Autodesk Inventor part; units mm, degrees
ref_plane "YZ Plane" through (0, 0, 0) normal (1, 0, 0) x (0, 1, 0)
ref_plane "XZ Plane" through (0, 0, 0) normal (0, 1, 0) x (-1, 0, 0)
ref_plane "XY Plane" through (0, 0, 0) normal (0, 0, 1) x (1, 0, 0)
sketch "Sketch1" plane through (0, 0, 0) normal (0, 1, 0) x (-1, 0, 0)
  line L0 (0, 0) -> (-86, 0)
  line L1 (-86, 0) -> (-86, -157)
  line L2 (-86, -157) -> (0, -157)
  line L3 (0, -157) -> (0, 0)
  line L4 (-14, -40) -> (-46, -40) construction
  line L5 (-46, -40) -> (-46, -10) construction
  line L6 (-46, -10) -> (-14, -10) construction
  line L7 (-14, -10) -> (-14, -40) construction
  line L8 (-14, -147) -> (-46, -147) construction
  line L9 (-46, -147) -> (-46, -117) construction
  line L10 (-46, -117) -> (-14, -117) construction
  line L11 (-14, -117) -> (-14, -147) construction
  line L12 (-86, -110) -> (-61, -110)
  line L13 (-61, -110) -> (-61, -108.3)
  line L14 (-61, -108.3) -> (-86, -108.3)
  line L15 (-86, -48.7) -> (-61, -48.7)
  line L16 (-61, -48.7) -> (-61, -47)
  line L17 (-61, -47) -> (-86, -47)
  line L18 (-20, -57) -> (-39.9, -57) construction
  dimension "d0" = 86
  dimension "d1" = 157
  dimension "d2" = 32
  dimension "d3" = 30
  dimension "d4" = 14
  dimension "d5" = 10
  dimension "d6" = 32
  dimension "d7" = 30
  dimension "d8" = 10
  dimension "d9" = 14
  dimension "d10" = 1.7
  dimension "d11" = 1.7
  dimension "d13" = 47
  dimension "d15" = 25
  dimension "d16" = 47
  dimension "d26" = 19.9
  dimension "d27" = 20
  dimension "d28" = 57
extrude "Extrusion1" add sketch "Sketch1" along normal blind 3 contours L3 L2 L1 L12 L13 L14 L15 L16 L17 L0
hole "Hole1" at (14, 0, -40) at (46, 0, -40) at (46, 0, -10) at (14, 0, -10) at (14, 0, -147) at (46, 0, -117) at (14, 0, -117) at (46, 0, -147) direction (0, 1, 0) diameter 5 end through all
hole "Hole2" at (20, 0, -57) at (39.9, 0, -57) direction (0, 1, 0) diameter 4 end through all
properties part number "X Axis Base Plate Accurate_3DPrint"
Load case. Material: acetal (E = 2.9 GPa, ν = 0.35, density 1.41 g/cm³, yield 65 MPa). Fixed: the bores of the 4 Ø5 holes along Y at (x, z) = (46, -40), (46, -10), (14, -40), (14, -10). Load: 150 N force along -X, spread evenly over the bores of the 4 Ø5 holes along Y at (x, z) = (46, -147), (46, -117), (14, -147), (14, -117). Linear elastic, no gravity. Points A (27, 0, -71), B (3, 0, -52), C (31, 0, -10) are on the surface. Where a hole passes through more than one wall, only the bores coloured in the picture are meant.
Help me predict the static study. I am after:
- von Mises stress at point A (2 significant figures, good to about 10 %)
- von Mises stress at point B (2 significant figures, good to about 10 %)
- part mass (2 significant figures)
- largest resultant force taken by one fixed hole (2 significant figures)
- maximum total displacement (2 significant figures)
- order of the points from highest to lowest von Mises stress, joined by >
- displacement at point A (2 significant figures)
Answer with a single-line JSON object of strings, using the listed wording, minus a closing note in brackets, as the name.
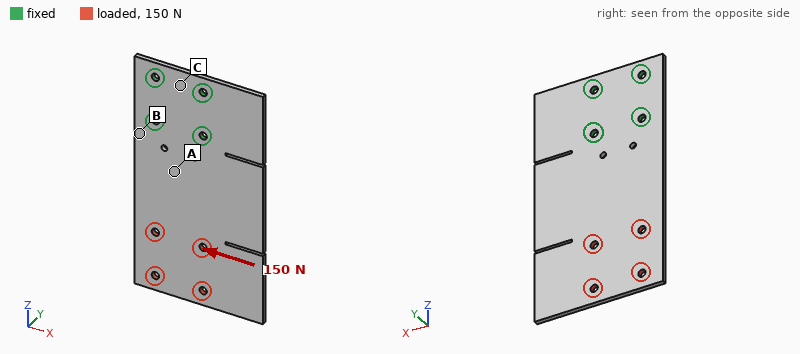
{"von Mises stress at point A": "2.3 MPa", "von Mises stress at point B": "4.6 MPa", "part mass": "56 g", "largest resultant force taken by one fixed hole": "290 N", "maximum total displacement": "0.50 mm", "order of the points from highest to lowest von Mises stress, joined by >": "B > A > C", "displacement at point A": "0.086 mm"}
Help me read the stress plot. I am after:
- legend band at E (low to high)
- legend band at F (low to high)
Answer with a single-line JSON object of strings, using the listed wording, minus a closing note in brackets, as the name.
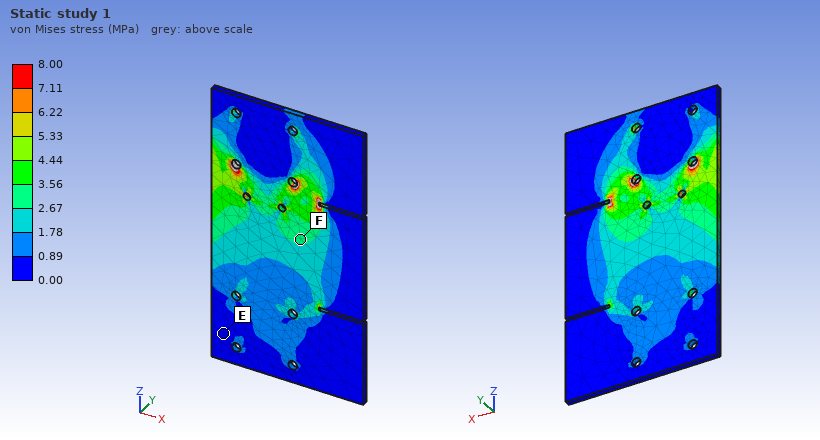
{"legend band at E": "0.00 to 0.89 MPa", "legend band at F": "2.67 to 3.56 MPa"}
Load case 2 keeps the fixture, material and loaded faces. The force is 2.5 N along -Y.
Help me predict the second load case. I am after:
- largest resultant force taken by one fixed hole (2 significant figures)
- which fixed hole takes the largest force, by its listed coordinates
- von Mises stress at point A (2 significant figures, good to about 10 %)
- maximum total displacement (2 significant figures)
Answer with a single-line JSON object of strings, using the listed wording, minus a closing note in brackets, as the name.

{"largest resultant force taken by one fixed hole": "2.6 N", "which fixed hole takes the largest force, by its listed coordinates": "(46, -40)", "von Mises stress at point A": "1.3 MPa", "maximum total displacement": "2.0 mm"}
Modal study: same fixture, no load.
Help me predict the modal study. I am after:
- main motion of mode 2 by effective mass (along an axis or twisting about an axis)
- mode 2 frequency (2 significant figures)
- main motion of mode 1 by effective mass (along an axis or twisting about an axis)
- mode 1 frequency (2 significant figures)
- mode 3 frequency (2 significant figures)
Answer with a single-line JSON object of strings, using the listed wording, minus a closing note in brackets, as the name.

{"main motion of mode 2 by effective mass": "twisting about Z", "mode 2 frequency": "130 Hz", "main motion of mode 1 by effective mass": "along Y", "mode 1 frequency": "47 Hz", "mode 3 frequency": "260 Hz"}
